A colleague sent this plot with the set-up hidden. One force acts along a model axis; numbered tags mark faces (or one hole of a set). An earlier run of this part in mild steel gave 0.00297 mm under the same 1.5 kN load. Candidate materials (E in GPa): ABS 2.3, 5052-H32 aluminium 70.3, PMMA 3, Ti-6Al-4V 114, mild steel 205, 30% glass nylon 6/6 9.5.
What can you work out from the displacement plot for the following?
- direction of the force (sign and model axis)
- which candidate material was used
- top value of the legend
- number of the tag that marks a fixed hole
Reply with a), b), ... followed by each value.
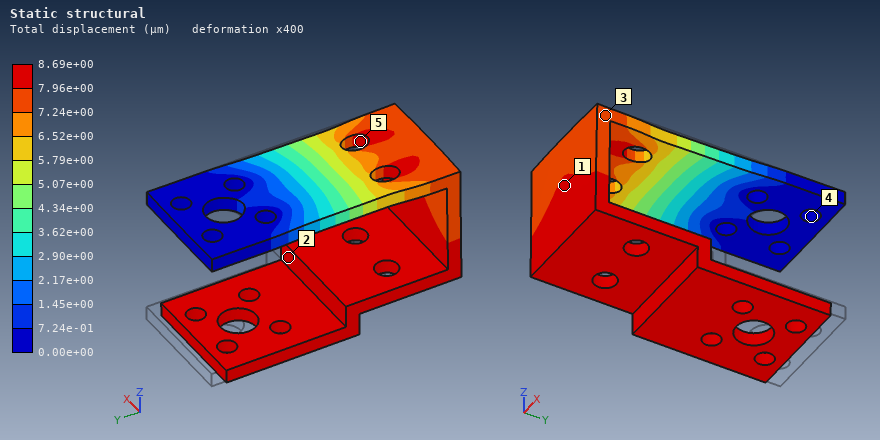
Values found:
a) -Y
b) 5052-H32 aluminium
c) 8.69e+00 µm
d) 4
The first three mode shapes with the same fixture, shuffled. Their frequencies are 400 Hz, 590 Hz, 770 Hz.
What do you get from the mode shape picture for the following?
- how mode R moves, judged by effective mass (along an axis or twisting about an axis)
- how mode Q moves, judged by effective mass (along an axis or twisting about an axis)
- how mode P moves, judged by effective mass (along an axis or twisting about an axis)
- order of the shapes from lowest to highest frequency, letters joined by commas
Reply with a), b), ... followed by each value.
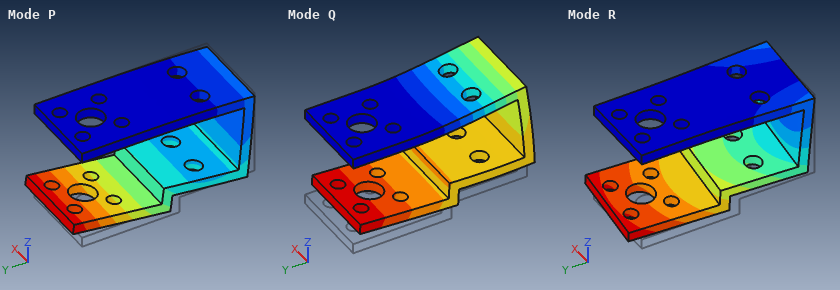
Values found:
a) along X
b) along Z
c) along Y
d) P, R, Q
